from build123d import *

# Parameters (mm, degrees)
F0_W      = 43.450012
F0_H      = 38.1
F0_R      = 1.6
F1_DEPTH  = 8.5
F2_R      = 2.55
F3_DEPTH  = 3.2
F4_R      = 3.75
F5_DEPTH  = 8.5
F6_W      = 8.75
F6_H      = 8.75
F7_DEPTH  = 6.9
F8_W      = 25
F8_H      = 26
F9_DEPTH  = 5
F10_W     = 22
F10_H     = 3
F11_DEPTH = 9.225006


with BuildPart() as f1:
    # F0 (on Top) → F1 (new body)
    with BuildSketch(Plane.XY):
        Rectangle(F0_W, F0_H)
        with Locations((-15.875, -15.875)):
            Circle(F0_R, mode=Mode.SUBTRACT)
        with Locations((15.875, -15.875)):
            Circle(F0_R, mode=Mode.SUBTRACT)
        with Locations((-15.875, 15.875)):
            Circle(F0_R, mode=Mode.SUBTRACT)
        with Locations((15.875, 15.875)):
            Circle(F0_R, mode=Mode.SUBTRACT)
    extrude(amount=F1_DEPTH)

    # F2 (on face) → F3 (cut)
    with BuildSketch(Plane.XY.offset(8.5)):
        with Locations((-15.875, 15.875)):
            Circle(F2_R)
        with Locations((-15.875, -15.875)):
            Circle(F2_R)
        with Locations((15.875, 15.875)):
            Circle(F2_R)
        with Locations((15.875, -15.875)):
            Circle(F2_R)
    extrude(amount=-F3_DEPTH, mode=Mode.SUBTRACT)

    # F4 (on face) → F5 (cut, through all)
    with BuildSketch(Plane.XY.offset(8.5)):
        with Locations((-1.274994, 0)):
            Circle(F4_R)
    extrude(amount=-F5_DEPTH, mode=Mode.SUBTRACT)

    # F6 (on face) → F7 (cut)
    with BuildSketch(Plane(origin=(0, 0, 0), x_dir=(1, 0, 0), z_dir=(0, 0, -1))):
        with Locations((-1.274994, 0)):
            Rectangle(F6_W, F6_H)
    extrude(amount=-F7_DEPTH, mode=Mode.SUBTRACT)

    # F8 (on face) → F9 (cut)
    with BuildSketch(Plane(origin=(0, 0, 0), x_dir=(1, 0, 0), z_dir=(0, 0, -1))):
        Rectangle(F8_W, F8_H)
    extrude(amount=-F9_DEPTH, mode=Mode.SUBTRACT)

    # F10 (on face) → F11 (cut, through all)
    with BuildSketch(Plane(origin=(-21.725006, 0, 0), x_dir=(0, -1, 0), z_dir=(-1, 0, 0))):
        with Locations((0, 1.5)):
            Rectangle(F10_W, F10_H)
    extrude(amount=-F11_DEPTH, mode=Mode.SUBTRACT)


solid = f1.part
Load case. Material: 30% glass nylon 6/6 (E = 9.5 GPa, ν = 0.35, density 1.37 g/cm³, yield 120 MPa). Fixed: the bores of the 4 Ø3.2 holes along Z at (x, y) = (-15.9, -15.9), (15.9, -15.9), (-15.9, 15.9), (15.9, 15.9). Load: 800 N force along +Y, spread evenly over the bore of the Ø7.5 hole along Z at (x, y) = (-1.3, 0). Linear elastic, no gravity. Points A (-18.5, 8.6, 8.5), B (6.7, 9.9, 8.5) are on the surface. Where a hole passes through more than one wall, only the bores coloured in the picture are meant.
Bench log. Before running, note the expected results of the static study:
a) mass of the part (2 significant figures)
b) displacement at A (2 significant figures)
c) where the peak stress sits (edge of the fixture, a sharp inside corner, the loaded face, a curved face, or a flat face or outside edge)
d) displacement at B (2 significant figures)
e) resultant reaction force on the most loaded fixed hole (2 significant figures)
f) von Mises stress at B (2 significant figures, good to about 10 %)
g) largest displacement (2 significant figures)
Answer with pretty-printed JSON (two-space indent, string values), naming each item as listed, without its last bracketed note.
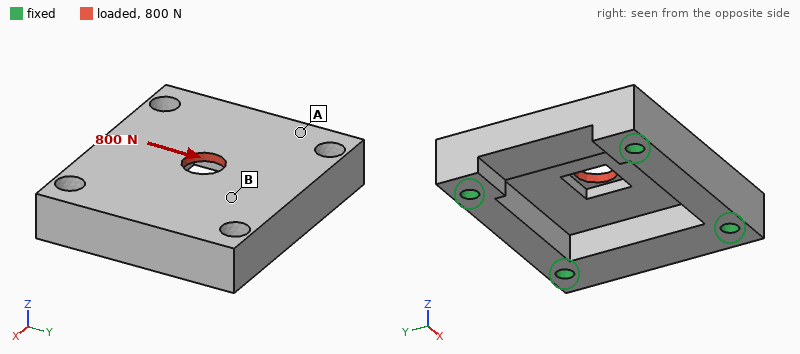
{
  "mass of the part": "13 g",
  "displacement at A": "4.1 µm",
  "where the peak stress sits": "the loaded face",
  "displacement at B": "9.8 µm",
  "resultant reaction force on the most loaded fixed hole": "230 N",
  "von Mises stress at B": "5.8 MPa",
  "largest displacement": "26 µm"
}
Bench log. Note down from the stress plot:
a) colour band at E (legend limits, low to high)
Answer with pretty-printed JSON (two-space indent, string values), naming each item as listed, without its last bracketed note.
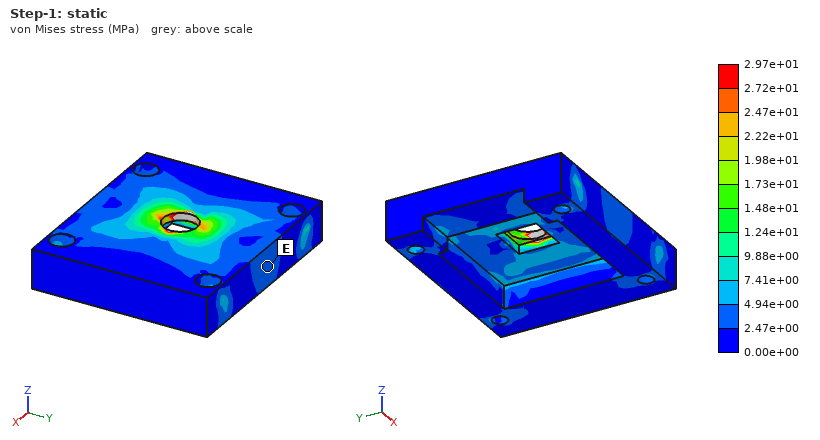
{
  "colour band at E": "2.47e+00 to 4.94e+00 MPa"
}
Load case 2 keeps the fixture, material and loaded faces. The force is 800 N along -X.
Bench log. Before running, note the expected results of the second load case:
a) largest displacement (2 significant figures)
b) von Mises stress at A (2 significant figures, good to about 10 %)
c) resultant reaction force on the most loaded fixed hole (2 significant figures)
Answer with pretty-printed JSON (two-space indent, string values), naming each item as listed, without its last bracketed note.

{
  "largest displacement": "26 µm",
  "von Mises stress at A": "2.6 MPa",
  "resultant reaction force on the most loaded fixed hole": "220 N"
}
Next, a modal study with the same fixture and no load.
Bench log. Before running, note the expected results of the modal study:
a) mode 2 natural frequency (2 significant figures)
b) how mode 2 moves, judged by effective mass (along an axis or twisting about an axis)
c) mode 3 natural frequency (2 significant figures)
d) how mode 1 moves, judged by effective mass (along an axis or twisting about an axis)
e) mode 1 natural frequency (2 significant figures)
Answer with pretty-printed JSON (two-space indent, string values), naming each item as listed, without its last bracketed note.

{
  "mode 2 natural frequency": "14 kHz",
  "how mode 2 moves, judged by effective mass": "twisting about Y",
  "mode 3 natural frequency": "14 kHz",
  "how mode 1 moves, judged by effective mass": "along Z",
  "mode 1 natural frequency": "10 kHz"
}
